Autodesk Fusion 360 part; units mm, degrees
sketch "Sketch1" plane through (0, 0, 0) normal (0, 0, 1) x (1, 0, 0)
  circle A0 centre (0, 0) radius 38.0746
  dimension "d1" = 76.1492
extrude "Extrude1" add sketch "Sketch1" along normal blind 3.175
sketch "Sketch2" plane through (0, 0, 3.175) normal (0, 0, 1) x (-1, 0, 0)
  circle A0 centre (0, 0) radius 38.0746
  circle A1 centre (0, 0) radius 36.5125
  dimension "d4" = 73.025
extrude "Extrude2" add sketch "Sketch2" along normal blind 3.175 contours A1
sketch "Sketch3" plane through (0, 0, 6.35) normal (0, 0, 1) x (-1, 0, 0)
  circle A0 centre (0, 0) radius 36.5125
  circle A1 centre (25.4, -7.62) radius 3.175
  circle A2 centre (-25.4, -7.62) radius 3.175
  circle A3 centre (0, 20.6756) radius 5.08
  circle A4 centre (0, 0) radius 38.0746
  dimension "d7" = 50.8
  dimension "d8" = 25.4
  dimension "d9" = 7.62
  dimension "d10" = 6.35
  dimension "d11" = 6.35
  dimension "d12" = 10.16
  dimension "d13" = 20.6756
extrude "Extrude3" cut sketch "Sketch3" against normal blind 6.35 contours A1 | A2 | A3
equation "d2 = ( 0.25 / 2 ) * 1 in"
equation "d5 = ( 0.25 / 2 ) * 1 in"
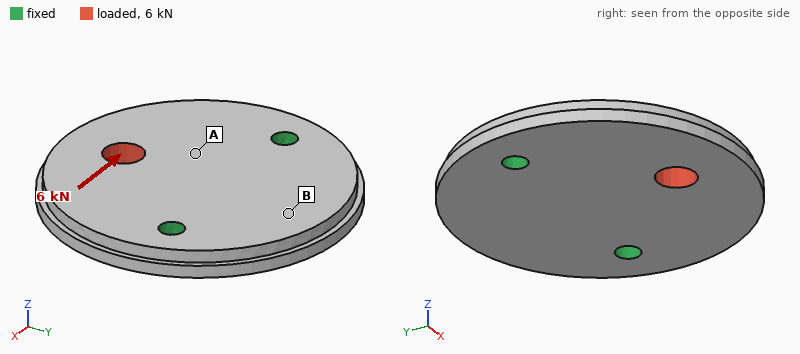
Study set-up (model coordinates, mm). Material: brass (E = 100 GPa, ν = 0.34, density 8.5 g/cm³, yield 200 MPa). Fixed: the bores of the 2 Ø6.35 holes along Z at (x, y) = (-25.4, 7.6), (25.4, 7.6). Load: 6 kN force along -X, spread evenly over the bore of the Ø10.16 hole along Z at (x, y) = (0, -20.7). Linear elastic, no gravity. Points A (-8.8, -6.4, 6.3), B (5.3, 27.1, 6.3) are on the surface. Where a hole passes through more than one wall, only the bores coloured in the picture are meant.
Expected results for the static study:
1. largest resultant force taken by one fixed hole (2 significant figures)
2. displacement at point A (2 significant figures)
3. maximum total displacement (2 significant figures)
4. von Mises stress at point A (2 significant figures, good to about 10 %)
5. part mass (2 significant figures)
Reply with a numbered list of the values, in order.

1. 4.3 kN
2. 7.5 µm
3. 21 µm
4. 30 MPa
5. 230 g
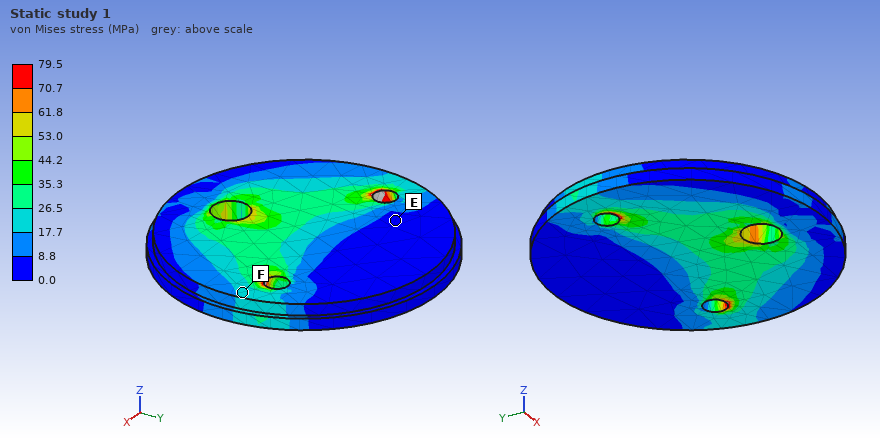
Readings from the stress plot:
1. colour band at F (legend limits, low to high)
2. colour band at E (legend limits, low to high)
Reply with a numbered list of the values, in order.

1. 17.7 to 26.5 MPa
2. 0.0 to 8.8 MPa
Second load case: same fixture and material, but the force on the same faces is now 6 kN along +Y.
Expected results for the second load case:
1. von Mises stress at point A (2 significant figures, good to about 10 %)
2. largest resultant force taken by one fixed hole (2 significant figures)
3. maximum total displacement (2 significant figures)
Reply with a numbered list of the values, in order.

1. 21 MPa
2. 3.1 kN
3. 12 µm
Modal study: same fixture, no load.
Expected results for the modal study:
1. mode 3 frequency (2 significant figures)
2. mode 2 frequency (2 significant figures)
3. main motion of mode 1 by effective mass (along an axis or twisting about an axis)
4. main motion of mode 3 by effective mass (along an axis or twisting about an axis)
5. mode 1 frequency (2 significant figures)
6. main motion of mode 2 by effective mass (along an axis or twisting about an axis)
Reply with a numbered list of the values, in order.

1. 4700 Hz
2. 4100 Hz
3. along Z
4. twisting about Y
5. 2000 Hz
6. along Z
